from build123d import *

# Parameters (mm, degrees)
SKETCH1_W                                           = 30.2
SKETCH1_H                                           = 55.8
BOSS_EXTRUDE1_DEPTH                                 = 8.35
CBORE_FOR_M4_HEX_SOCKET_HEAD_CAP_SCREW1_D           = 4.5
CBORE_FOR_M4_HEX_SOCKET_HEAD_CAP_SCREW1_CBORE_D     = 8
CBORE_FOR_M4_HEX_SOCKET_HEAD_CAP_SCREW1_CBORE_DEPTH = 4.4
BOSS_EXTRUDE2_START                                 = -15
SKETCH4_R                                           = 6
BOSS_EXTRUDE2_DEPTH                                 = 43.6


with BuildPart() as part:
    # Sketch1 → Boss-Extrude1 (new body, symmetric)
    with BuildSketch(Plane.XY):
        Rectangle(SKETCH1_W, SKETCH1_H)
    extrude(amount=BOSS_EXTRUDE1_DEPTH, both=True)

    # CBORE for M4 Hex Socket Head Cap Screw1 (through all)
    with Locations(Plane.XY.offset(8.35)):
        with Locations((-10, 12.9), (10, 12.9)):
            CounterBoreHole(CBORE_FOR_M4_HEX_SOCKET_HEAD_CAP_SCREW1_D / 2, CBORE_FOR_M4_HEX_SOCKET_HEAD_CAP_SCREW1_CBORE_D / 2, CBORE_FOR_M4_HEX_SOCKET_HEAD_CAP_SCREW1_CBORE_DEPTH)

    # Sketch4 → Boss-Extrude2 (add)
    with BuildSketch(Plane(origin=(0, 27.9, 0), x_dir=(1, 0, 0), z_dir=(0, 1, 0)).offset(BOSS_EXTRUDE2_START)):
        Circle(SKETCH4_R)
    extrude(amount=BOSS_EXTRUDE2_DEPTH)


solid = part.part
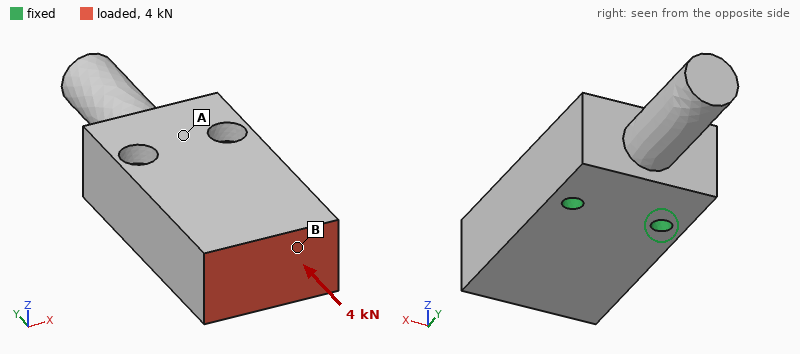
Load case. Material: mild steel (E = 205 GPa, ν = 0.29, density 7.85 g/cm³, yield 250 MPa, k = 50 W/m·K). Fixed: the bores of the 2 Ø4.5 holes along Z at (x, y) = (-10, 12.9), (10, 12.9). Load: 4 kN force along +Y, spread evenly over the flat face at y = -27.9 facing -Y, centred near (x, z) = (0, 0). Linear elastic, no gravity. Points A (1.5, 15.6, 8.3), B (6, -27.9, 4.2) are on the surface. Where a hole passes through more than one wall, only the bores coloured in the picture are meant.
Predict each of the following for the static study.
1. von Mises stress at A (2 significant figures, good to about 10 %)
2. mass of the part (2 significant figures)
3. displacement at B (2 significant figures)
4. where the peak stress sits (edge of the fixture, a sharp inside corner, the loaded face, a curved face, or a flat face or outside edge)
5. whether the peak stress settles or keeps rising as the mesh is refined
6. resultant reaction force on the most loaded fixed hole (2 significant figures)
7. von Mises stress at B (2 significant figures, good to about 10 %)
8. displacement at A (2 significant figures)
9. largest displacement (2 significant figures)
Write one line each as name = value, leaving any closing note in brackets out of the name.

von Mises stress at A = 3.7 MPa
mass of the part = 240 g
displacement at B = 2.6 µm
where the peak stress sits = edge of the fixture
whether the peak stress settles or keeps rising as the mesh is refined = keeps rising
resultant reaction force on the most loaded fixed hole = 2.0 kN
von Mises stress at B = 7.9 MPa
displacement at A = 0.61 µm
largest displacement = 2.8 µm
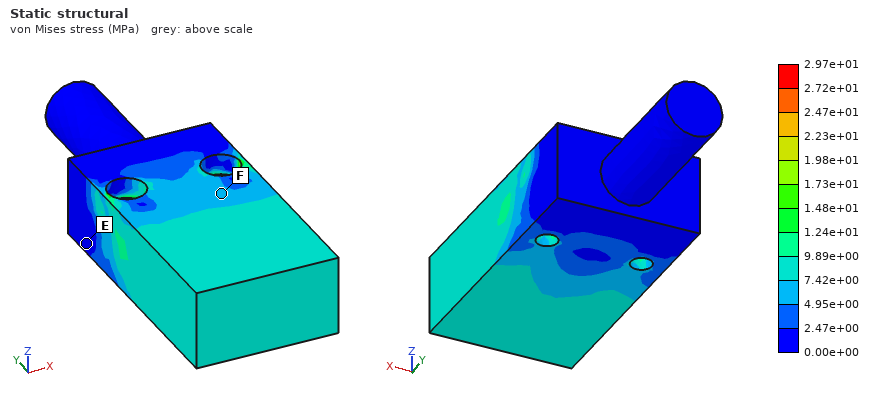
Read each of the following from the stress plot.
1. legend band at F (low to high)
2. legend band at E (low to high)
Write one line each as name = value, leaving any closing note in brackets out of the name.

legend band at F = 4.95e+00 to 7.42e+00 MPa
legend band at E = 0.00e+00 to 2.47e+00 MPa
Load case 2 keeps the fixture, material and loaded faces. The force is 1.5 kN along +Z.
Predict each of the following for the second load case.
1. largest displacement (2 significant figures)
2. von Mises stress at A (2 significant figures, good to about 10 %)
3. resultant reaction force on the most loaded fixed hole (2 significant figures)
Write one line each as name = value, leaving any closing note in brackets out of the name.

largest displacement = 24 µm
von Mises stress at A = 17 MPa
resultant reaction force on the most loaded fixed hole = 780 N
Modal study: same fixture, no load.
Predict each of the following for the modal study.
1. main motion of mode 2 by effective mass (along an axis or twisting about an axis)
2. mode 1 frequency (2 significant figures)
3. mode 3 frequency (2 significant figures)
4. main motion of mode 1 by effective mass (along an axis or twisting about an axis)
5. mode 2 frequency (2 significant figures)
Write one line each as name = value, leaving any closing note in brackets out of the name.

main motion of mode 2 by effective mass = along Z
mode 1 frequency = 5700 Hz
mode 3 frequency = 8000 Hz
main motion of mode 1 by effective mass = along Z
mode 2 frequency = 7300 Hz
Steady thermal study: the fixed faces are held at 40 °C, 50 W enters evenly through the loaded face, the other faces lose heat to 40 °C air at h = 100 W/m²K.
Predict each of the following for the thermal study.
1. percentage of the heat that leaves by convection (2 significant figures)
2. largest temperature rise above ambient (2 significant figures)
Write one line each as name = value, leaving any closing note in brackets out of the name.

percentage of the heat that leaves by convection = 27 %
largest temperature rise above ambient = 70 K
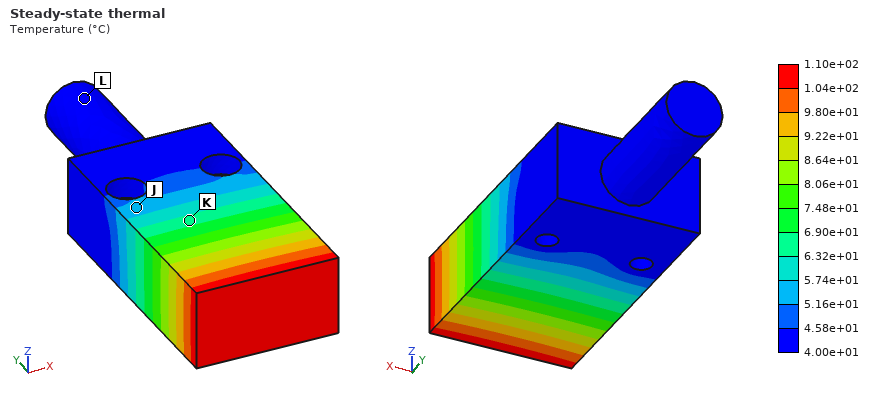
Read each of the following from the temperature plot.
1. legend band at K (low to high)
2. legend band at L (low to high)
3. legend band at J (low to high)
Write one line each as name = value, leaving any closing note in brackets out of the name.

legend band at K = 6.32e+01 to 6.90e+01 °C
legend band at L = 4.00e+01 to 4.58e+01 °C
legend band at J = 5.16e+01 to 5.74e+01 °C
